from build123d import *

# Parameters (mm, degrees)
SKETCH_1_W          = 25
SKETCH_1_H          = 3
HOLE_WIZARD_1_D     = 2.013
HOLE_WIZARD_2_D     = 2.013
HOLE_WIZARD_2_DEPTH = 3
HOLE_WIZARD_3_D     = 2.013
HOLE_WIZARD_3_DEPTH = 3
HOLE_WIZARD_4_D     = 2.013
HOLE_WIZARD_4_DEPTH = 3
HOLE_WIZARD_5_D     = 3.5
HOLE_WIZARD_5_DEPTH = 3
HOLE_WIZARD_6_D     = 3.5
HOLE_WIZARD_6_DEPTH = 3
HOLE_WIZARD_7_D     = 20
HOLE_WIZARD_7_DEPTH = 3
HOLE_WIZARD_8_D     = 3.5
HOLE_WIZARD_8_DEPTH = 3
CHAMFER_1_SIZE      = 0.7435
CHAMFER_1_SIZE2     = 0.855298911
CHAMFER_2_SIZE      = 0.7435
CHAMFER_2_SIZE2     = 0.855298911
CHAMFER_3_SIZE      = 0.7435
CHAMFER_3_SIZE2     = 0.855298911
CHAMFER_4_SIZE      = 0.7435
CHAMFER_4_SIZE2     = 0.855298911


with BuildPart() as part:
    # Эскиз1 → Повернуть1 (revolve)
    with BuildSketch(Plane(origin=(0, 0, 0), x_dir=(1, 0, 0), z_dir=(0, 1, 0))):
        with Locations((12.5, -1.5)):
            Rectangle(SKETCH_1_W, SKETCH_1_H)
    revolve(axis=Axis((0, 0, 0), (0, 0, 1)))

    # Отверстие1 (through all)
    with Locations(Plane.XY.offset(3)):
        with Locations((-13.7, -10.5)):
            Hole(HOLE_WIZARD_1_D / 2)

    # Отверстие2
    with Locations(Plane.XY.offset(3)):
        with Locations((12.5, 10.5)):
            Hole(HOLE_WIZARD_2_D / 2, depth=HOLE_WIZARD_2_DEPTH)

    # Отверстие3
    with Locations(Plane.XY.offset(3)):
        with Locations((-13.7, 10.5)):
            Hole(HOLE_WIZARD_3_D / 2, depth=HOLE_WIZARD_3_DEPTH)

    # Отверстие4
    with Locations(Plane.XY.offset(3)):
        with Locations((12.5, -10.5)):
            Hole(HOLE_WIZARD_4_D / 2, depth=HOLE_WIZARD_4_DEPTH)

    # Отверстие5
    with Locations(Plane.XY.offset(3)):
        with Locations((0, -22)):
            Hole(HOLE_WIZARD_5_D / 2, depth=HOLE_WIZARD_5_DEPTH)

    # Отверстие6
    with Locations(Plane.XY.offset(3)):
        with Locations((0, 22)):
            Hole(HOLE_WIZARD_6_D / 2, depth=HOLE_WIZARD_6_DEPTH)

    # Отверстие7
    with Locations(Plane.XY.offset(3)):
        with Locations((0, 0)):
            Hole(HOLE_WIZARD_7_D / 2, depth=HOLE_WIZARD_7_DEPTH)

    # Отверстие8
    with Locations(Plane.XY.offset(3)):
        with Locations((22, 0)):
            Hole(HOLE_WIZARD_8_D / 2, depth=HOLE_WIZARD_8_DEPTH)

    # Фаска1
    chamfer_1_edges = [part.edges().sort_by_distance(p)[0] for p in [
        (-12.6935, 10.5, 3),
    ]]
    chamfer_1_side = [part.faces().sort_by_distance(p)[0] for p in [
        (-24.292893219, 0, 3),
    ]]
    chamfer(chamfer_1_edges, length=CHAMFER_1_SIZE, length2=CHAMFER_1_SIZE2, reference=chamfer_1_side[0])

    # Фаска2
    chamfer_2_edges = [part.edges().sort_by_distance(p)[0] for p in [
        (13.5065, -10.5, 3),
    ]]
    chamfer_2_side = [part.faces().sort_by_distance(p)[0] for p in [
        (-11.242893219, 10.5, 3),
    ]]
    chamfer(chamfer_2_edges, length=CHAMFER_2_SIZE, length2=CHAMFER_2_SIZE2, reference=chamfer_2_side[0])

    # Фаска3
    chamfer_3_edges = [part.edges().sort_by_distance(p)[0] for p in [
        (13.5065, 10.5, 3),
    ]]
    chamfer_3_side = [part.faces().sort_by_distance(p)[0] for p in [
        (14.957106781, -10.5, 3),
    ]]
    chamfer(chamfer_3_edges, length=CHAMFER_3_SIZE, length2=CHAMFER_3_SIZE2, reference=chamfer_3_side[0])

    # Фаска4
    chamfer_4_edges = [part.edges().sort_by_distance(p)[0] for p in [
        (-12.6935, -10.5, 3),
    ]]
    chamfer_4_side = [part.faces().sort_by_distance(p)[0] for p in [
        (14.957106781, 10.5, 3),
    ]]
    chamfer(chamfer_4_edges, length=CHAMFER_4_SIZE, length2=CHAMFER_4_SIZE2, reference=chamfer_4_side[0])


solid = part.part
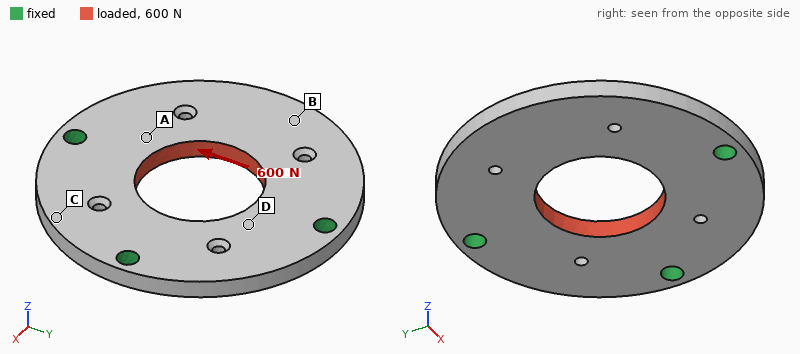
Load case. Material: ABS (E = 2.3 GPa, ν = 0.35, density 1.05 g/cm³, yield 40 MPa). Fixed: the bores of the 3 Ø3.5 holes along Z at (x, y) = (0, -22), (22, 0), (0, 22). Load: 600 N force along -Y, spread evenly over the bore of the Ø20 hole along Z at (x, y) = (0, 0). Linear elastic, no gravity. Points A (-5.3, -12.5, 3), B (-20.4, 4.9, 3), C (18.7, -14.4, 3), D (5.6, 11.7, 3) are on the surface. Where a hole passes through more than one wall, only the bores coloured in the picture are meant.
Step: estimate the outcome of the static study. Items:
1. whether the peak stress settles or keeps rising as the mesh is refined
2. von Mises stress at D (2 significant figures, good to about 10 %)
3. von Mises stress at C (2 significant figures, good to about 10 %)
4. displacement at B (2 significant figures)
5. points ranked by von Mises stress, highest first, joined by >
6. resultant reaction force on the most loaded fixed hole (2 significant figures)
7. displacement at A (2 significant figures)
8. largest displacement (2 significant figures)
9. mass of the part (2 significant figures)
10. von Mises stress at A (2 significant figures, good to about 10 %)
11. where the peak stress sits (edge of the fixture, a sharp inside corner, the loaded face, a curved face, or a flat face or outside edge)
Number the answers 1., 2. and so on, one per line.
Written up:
1. keeps rising
2. 4.8 MPa
3. 2.2 MPa
4. 51 µm
5. A > D > C > B
6. 240 N
7. 40 µm
8. 71 µm
9. 5.1 g
10. 6.5 MPa
11. edge of the fixture
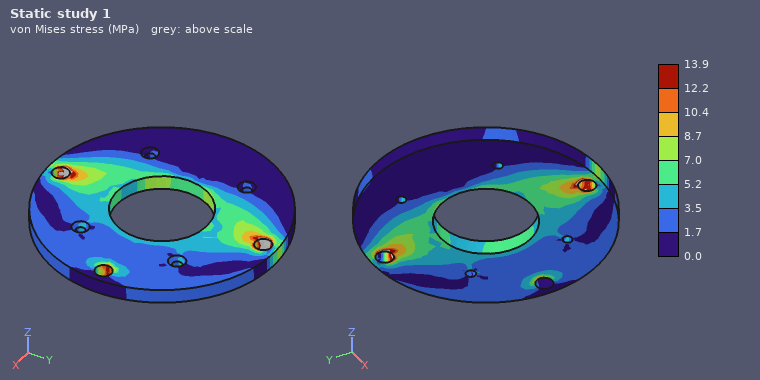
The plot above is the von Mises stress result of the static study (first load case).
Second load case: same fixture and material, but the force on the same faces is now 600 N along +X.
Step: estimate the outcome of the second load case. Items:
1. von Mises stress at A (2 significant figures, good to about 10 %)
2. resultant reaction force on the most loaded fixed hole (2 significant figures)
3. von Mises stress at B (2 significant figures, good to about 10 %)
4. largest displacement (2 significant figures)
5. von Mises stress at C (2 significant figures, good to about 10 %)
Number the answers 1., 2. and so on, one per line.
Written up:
1. 4.6 MPa
2. 210 N
3. 3.3 MPa
4. 75 µm
5. 2.3 MPa
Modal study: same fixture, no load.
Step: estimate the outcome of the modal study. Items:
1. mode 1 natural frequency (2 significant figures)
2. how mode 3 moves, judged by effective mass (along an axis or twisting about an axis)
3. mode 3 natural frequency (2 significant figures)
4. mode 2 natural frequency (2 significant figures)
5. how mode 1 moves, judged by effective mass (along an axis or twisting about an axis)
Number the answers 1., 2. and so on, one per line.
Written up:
1. 1000 Hz
2. along Z
3. 4000 Hz
4. 2800 Hz
5. along Z
